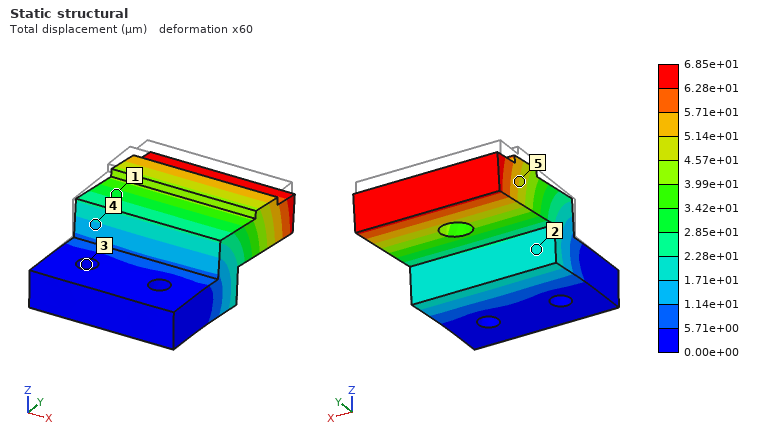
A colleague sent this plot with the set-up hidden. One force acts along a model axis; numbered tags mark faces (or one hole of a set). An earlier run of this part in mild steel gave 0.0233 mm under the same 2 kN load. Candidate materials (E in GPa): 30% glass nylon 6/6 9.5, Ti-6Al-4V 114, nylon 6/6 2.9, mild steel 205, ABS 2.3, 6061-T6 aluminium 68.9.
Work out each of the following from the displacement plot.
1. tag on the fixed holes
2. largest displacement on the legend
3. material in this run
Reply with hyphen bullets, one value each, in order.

- 3
- 6.85e+01 µm
- 6061-T6 aluminium
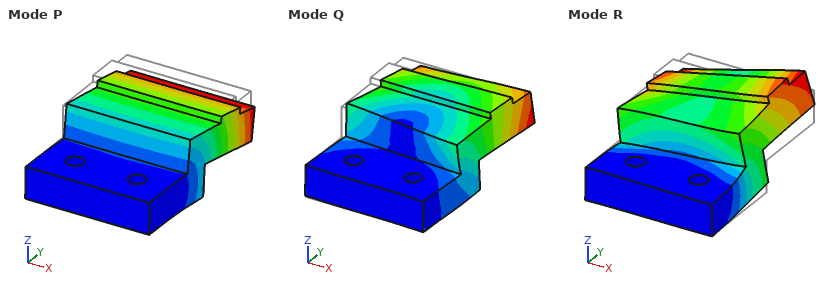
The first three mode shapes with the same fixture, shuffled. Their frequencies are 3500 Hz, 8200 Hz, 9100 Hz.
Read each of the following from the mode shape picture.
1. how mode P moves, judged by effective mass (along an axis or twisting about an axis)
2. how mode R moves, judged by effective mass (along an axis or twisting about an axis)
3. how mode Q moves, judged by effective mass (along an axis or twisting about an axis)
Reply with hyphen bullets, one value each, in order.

- along Z
- along X
- along X
